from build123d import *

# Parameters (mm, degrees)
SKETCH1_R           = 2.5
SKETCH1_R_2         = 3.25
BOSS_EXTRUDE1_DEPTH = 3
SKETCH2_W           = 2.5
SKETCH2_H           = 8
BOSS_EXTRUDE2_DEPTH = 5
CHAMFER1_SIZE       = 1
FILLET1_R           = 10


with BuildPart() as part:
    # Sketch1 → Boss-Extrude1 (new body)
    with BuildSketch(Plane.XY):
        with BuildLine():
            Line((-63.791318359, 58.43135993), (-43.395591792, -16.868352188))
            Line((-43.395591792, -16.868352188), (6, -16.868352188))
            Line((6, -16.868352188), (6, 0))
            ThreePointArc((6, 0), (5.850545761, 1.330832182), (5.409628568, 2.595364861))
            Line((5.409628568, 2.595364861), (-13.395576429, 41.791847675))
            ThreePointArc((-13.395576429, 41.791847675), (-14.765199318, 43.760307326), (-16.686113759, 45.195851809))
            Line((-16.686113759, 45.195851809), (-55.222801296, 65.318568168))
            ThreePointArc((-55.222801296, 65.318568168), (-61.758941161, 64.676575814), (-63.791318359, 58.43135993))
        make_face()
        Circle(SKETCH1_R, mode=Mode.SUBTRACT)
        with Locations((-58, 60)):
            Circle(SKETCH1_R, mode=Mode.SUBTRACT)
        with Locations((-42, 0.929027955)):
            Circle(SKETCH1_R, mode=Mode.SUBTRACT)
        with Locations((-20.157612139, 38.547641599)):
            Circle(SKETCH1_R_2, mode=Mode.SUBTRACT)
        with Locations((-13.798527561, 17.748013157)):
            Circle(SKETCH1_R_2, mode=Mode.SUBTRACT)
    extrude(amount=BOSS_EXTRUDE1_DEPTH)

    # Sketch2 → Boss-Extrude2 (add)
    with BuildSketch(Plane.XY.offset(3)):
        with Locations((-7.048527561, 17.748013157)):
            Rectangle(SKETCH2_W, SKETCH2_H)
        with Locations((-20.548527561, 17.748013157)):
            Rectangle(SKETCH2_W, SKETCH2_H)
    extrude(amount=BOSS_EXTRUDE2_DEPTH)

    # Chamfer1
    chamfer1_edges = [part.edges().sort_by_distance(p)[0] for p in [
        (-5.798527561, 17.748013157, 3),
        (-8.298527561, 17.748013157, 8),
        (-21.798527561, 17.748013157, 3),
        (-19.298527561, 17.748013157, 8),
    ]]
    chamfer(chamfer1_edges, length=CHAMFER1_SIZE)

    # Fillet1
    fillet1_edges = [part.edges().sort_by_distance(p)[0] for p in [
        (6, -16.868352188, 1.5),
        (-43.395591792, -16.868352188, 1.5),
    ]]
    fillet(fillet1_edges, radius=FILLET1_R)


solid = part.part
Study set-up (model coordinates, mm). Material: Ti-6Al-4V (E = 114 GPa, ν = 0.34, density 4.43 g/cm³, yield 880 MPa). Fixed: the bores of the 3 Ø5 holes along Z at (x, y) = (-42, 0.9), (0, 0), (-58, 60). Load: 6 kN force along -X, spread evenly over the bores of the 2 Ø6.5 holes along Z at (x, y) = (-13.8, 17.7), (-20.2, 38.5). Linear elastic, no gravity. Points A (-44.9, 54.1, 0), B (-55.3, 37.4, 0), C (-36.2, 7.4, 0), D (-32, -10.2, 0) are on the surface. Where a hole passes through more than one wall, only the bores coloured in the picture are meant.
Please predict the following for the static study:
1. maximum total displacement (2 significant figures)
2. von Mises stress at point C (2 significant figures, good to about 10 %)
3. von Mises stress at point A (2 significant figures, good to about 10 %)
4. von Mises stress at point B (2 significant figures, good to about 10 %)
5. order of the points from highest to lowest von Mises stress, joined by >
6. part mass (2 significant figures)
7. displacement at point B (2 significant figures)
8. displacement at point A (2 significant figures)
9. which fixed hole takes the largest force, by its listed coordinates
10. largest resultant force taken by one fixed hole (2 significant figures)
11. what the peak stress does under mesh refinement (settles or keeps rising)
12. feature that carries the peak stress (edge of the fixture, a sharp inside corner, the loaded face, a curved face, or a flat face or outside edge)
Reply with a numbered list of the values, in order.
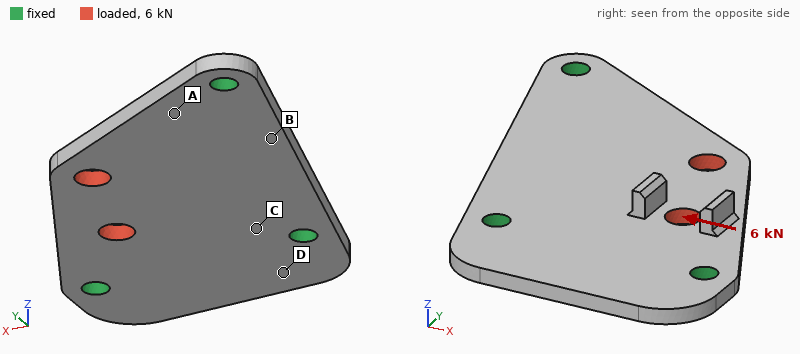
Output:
1. 26 µm
2. 70 MPa
3. 53 MPa
4. 21 MPa
5. C > A > B > D
6. 47 g
7. 16 µm
8. 10 µm
9. (-42, 0.9)
10. 2.9 kN
11. keeps rising
12. edge of the fixture
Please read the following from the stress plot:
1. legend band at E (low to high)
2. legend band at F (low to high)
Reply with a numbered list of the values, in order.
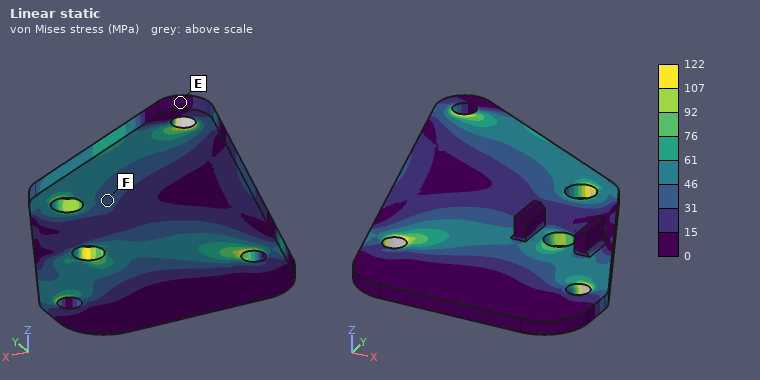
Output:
1. 0 to 15 MPa
2. 31 to 46 MPa
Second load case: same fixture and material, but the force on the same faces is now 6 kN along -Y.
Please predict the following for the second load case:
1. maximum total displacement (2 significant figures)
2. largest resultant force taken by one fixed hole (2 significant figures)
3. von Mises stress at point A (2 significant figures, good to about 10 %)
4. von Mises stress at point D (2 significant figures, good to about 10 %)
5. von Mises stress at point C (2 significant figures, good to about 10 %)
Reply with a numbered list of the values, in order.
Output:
1. 23 µm
2. 2.8 kN
3. 25 MPa
4. 19 MPa
5. 61 MPa
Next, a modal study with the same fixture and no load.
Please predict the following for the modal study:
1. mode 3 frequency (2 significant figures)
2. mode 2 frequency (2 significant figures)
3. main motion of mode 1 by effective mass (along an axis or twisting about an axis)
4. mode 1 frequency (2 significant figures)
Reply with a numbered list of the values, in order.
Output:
1. 6400 Hz
2. 5100 Hz
3. along Z
4. 2400 Hz
